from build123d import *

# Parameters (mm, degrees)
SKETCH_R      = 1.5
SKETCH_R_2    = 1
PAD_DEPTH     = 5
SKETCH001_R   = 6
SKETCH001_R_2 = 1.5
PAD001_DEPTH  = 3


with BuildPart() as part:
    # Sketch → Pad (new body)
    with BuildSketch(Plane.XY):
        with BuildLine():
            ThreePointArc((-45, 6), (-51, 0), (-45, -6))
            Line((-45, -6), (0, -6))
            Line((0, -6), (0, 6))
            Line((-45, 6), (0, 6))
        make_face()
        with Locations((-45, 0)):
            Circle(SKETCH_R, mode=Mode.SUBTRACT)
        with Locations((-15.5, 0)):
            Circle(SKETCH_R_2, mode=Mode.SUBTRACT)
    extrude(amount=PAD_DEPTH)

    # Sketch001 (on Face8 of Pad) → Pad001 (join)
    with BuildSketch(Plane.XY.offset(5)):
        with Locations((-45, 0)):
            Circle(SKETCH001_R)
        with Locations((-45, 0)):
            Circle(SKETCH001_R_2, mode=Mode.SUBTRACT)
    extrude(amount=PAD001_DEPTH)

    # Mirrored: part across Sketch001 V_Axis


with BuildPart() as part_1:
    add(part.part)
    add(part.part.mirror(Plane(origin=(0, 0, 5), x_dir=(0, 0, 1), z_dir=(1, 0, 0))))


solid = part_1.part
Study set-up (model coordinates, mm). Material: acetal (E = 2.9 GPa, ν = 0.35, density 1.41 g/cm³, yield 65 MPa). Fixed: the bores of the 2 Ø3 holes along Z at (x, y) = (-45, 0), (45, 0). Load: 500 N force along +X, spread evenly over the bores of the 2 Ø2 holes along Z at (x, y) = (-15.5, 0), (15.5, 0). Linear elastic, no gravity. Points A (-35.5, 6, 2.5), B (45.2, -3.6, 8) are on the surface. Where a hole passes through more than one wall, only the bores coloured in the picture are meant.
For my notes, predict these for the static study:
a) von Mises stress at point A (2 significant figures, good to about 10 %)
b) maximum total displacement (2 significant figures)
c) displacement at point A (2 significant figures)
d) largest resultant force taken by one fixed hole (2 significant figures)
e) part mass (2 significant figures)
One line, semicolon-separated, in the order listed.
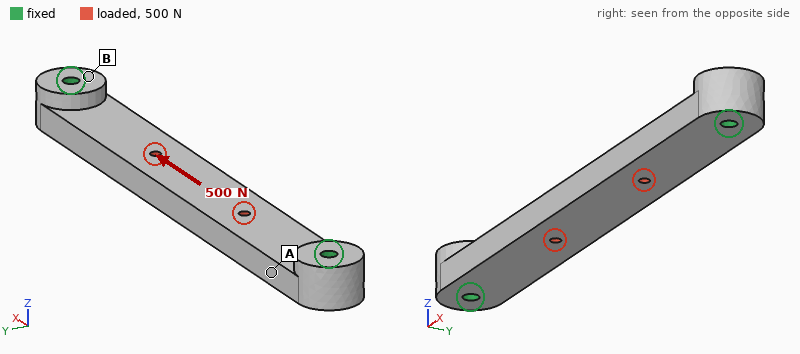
3.9 MPa; 53 µm; 17 µm; 250 N; 9.2 g
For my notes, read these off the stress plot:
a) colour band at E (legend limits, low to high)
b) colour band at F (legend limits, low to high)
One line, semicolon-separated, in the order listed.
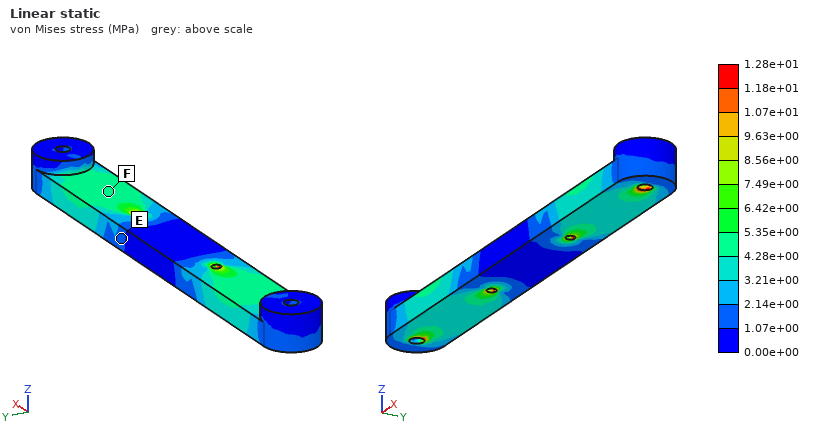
1.07e+00 to 2.14e+00 MPa; 4.28e+00 to 5.35e+00 MPa
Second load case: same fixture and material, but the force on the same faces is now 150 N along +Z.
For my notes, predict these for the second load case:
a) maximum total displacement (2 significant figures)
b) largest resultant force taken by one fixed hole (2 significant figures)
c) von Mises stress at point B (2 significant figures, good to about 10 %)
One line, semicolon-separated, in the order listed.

0.96 mm; 80 N; 4.8 MPa
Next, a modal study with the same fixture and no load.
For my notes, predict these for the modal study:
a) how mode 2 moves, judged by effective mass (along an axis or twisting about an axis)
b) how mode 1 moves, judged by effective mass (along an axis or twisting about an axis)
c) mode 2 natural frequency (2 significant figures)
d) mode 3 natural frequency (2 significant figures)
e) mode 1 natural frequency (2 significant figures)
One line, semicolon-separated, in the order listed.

along Y; along Z; 1700 Hz; 2600 Hz; 1000 Hz
